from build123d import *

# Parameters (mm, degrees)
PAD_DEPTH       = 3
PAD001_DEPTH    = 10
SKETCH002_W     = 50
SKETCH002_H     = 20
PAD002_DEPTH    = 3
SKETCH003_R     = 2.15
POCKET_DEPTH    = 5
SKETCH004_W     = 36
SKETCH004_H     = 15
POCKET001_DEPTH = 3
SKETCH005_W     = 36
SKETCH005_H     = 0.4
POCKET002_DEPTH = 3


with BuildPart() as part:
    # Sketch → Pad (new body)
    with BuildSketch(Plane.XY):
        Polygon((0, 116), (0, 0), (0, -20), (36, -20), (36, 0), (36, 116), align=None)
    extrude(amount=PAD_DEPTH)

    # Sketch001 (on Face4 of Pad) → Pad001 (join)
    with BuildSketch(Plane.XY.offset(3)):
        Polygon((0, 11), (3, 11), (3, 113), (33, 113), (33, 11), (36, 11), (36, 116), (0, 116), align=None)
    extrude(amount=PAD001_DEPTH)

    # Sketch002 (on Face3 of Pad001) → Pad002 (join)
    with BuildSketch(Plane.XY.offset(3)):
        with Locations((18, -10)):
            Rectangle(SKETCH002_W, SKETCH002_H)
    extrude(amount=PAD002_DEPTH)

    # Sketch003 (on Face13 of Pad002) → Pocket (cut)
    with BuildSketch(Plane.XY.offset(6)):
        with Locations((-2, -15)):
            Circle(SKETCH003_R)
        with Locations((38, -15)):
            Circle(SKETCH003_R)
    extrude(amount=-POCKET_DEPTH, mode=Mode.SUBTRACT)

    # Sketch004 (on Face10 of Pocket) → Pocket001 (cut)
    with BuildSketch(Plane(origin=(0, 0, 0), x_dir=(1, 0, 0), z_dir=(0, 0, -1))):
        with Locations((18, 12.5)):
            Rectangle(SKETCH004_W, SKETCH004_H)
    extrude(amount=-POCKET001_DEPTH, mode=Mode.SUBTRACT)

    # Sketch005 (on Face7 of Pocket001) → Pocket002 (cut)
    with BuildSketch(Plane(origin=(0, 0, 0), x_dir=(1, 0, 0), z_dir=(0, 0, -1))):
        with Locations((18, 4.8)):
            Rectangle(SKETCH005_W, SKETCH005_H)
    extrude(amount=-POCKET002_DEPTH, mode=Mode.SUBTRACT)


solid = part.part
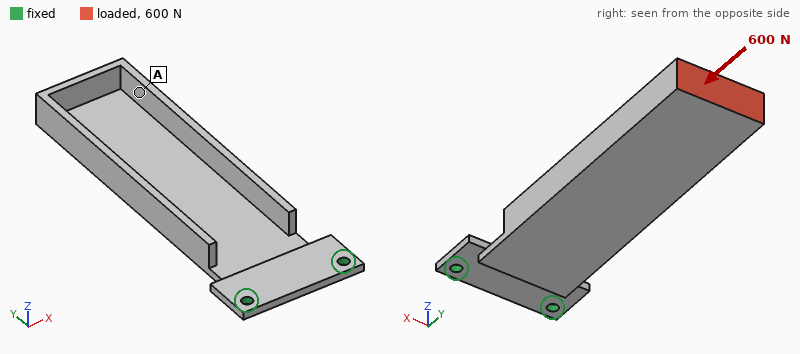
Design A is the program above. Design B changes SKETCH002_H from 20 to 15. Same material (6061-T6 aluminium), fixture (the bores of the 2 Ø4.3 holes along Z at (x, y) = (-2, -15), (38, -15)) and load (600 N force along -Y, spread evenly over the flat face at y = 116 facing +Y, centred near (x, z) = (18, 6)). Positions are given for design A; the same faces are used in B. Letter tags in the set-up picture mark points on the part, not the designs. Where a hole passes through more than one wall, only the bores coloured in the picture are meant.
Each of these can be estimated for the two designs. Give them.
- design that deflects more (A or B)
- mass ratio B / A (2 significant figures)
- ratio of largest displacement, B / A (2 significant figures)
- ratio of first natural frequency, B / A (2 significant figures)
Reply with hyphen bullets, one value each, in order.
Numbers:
- B
- 0.97
- 1.3
- 0.88
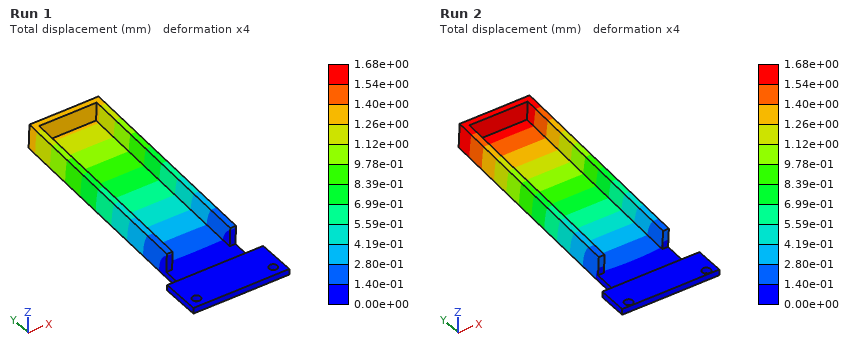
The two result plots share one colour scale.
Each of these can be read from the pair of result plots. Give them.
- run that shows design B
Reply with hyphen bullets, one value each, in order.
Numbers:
- Run 2
